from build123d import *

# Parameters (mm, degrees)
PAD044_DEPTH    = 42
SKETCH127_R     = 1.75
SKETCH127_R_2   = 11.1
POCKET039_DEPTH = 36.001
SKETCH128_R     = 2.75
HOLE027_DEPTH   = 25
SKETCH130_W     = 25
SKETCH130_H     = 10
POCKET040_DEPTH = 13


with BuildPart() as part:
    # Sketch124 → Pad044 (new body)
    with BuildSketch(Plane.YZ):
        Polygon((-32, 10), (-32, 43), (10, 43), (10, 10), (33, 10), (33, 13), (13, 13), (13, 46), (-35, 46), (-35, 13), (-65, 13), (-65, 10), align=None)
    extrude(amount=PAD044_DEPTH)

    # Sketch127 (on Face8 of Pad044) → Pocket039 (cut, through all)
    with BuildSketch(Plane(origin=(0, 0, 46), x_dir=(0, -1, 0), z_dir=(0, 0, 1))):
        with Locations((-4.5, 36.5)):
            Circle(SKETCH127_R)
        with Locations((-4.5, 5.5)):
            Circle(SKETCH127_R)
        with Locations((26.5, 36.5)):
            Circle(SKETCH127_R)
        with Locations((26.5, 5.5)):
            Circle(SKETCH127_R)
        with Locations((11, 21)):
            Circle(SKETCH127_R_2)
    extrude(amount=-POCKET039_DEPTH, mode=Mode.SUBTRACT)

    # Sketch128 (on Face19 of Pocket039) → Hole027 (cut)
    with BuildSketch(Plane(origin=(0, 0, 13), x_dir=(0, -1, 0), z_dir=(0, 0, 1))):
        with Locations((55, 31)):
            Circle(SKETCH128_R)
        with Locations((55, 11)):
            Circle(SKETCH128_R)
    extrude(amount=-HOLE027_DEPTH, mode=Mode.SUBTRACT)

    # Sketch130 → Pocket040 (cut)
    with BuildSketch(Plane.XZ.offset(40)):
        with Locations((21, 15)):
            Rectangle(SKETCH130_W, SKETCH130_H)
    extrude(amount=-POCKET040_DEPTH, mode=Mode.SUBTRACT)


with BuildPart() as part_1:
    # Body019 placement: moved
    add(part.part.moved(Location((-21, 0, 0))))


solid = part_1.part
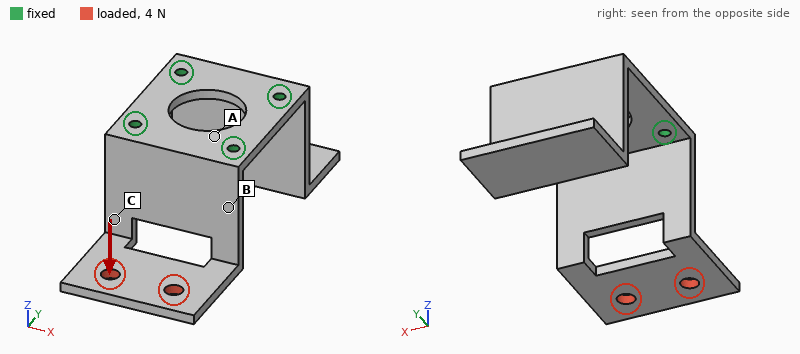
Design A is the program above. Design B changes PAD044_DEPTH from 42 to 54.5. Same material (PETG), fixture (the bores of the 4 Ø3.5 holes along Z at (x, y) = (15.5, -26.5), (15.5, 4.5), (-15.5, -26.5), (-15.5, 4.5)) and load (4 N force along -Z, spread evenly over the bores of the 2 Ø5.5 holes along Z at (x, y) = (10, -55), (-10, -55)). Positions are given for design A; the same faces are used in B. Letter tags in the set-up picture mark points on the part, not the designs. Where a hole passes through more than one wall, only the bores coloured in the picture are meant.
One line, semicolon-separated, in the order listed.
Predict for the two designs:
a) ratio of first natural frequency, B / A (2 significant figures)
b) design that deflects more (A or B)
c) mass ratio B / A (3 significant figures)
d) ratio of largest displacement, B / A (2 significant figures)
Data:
1.0; A; 1.34; 0.71
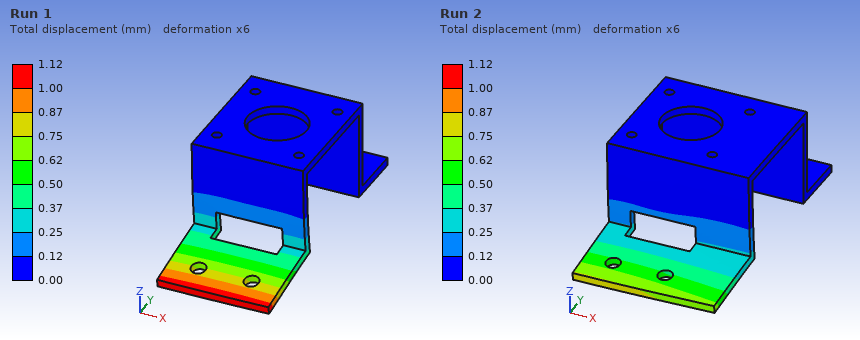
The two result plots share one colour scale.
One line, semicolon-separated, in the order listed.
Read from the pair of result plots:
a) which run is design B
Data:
Run 2
